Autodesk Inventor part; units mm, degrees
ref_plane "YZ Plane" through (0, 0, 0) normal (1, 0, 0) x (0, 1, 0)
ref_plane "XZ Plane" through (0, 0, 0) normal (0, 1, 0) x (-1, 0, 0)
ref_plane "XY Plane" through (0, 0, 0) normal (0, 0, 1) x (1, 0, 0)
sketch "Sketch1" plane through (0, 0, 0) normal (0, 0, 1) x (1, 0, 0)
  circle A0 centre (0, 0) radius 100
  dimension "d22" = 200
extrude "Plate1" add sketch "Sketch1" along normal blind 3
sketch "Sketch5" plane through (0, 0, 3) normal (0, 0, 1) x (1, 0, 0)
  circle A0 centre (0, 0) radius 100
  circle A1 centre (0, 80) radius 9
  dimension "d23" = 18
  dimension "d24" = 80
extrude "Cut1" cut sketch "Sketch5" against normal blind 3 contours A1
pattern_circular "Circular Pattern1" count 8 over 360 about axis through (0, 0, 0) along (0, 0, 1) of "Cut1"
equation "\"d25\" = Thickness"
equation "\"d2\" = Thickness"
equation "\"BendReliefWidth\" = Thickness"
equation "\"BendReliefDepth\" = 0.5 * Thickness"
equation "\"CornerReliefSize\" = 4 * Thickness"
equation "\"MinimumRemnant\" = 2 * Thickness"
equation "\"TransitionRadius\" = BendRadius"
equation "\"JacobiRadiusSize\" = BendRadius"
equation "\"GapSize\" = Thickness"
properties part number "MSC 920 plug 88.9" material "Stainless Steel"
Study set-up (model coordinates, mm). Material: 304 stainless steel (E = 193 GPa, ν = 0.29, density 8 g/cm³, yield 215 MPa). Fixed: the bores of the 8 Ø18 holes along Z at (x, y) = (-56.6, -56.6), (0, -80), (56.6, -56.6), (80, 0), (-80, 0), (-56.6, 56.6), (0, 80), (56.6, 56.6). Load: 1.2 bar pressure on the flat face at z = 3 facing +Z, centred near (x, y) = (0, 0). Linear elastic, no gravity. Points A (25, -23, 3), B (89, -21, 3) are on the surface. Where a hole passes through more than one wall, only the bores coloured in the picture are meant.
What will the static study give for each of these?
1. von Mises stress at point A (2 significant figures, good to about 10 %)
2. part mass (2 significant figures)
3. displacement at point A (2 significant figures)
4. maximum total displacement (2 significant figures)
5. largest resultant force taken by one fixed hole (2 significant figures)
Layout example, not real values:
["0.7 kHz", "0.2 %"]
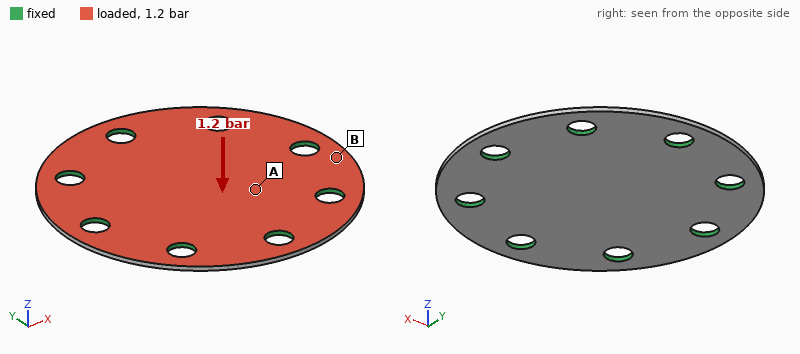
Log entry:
["21 MPa", "710 g", "0.079 mm", "0.12 mm", "440 N"]
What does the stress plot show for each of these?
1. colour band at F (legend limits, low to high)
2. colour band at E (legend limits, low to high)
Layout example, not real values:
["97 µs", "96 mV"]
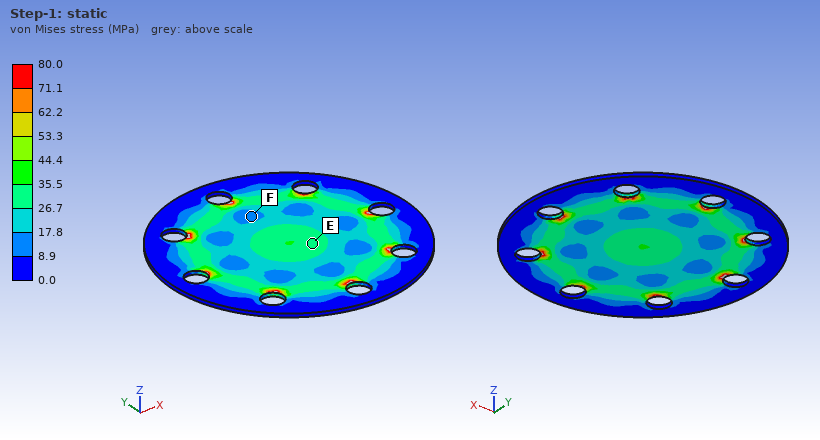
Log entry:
["8.9 to 17.8 MPa", "26.7 to 35.5 MPa"]
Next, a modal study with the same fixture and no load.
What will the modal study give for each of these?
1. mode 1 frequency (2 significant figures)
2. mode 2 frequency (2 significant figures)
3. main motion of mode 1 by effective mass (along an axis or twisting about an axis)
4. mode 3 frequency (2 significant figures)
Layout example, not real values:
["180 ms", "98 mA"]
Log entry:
["1300 Hz", "2600 Hz", "along Z", "2600 Hz"]
